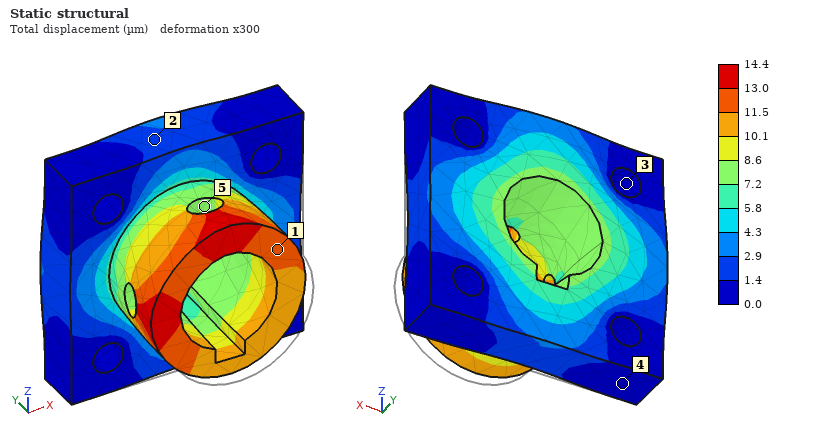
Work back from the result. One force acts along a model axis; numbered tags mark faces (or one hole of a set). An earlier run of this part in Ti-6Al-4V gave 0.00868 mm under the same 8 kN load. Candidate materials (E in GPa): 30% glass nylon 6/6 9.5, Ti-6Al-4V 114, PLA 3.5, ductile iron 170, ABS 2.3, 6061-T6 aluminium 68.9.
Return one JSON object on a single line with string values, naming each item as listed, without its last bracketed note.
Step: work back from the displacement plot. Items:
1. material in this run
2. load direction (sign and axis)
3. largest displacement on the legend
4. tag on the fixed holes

{"material in this run": "6061-T6 aluminium", "load direction": "+Y", "largest displacement on the legend": "14.4 µm", "tag on the fixed holes": "3"}
